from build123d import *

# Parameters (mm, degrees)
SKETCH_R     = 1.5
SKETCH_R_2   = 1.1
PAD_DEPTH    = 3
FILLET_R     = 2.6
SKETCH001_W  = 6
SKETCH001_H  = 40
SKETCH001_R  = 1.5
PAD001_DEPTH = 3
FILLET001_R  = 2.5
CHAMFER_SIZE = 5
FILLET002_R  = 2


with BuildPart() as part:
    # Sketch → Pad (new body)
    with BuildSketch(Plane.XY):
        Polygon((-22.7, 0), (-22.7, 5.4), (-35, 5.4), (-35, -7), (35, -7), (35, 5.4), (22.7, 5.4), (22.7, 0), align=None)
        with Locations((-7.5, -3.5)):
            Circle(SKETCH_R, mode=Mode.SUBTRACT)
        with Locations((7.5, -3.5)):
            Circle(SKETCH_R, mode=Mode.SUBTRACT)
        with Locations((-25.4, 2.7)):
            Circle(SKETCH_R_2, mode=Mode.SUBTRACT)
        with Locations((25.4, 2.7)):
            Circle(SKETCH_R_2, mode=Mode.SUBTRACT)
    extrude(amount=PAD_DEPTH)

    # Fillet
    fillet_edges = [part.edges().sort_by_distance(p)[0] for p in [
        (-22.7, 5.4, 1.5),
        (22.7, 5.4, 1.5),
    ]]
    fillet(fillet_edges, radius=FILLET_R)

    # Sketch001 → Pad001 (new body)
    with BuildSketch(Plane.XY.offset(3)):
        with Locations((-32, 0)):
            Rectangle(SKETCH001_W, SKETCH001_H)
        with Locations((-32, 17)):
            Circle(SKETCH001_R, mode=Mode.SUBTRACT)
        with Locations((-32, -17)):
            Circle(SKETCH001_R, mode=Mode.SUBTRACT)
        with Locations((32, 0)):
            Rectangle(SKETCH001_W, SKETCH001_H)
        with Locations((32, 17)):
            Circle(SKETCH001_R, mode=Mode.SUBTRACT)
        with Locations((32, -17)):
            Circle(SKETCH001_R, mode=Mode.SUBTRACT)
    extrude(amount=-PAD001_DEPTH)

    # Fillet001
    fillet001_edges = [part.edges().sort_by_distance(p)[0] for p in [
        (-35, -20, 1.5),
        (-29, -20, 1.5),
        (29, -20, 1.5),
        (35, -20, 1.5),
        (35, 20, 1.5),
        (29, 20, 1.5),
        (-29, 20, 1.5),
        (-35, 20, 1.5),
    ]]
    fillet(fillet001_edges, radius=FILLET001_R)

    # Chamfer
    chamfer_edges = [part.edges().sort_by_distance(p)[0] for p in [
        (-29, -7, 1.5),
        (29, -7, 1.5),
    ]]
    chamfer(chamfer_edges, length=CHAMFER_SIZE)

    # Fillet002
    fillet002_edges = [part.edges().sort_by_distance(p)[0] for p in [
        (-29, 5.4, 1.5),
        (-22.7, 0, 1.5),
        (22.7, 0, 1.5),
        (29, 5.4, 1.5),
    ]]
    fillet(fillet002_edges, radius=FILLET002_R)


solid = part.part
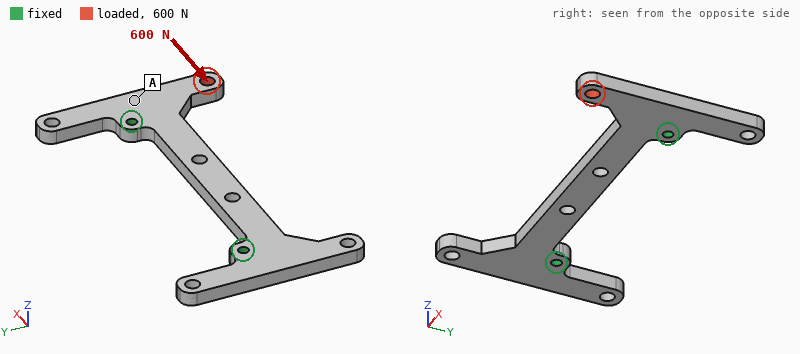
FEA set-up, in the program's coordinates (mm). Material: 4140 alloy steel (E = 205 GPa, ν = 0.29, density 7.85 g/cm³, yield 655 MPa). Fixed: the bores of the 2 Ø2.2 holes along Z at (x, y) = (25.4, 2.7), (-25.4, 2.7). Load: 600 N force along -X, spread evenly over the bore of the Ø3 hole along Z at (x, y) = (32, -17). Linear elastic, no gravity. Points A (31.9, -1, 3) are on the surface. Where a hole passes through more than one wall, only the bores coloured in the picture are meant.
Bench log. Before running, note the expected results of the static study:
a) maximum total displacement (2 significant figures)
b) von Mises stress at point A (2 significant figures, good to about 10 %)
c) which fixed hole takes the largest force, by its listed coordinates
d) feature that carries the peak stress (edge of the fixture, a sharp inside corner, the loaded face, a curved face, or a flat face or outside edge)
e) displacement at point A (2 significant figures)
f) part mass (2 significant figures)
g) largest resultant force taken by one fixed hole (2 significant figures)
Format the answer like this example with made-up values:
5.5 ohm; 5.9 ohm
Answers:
74 µm; 55 MPa; (-25.4, 2.7); edge of the fixture; 14 µm; 22 g; 580 N
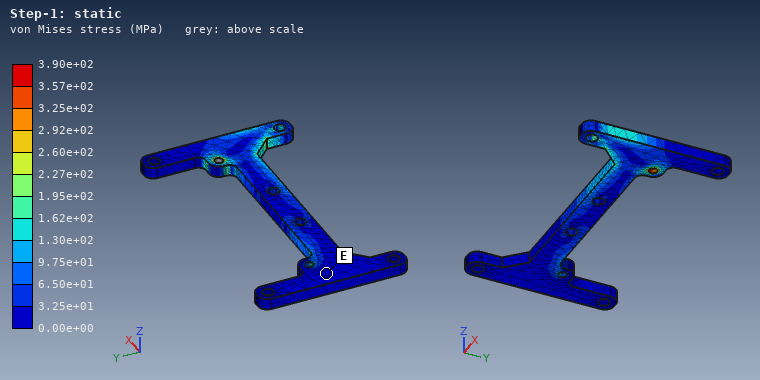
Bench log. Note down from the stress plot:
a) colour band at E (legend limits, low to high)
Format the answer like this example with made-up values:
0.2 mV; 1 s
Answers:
0.00e+00 to 3.25e+01 MPa
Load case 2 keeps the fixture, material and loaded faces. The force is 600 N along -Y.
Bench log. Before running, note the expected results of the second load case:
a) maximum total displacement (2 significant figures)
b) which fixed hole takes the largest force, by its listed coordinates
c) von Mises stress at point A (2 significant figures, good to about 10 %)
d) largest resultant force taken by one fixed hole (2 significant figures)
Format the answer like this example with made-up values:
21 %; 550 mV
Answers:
19 µm; (25.4, 2.7); 28 MPa; 660 N
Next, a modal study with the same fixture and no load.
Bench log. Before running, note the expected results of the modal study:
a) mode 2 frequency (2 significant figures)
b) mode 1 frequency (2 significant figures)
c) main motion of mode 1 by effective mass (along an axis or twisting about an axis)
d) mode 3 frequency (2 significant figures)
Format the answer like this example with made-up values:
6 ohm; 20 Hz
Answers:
5700 Hz; 5100 Hz; along Z; 5900 Hz
